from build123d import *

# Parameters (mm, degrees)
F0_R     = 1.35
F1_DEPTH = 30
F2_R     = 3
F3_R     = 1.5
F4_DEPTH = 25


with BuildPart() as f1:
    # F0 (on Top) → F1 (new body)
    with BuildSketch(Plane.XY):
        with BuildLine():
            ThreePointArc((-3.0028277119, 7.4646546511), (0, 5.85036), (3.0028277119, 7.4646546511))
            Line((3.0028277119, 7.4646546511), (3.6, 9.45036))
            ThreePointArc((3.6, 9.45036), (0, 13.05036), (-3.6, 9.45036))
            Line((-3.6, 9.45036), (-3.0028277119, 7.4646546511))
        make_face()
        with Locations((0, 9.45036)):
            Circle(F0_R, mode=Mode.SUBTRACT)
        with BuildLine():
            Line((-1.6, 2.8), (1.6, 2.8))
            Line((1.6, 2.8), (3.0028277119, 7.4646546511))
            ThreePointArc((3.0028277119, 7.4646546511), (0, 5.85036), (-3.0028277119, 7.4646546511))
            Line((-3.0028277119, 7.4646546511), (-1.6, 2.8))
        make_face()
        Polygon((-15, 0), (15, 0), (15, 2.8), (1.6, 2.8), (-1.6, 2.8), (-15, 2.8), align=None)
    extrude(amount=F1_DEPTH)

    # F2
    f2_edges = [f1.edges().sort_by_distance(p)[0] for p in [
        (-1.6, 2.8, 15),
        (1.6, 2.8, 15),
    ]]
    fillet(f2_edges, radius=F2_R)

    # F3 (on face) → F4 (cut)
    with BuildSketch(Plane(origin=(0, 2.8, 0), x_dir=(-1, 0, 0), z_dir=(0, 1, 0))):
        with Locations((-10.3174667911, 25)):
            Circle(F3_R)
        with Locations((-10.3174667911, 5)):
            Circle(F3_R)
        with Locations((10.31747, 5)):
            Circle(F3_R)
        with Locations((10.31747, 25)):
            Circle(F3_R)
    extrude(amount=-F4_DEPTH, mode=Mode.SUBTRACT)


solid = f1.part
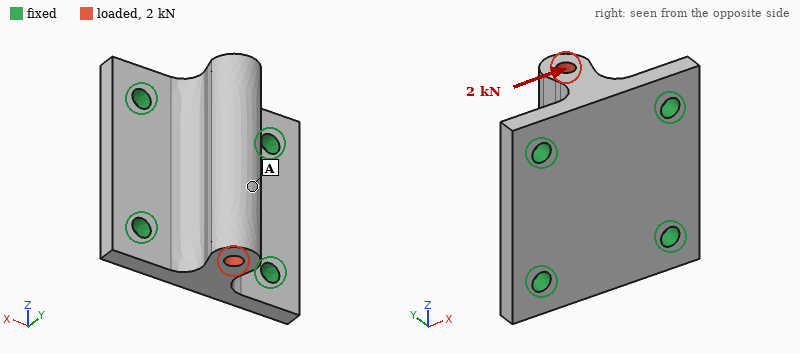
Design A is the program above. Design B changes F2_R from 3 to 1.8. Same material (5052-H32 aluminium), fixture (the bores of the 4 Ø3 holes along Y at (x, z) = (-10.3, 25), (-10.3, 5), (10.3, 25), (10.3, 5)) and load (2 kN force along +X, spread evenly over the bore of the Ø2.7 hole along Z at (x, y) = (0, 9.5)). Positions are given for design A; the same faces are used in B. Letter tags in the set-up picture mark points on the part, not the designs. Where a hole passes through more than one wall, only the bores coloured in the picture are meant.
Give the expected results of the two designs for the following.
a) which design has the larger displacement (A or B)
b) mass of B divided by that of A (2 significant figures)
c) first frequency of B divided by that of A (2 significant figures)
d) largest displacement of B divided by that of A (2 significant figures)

B
0.97
0.91
1.5
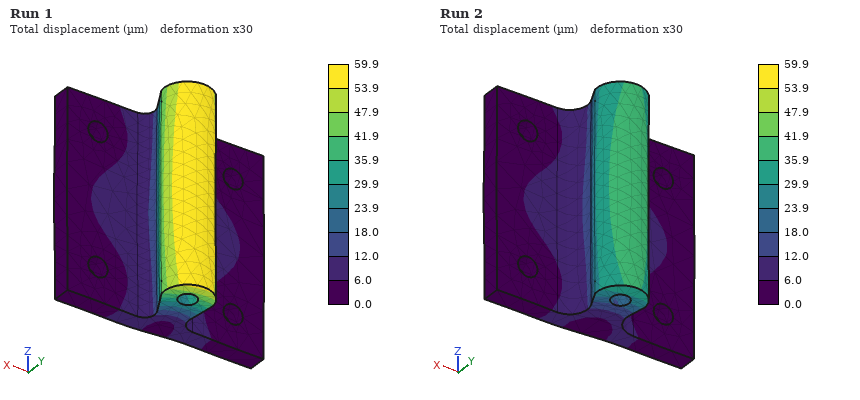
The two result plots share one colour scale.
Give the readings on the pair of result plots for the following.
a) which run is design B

Run 1
